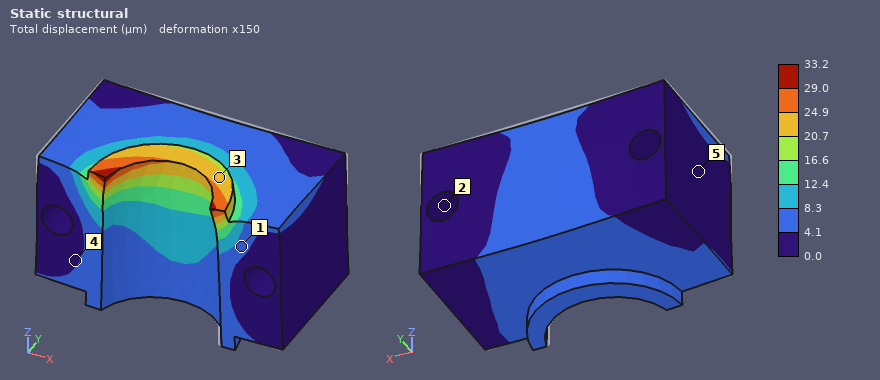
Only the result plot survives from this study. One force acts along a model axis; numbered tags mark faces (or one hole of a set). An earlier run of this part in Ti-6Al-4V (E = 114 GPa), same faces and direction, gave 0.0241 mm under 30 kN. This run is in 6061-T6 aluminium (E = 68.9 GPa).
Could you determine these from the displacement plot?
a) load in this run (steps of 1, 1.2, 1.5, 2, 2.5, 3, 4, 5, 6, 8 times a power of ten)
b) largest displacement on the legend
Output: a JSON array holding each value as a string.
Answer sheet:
["25 kN", "33.2 µm"]
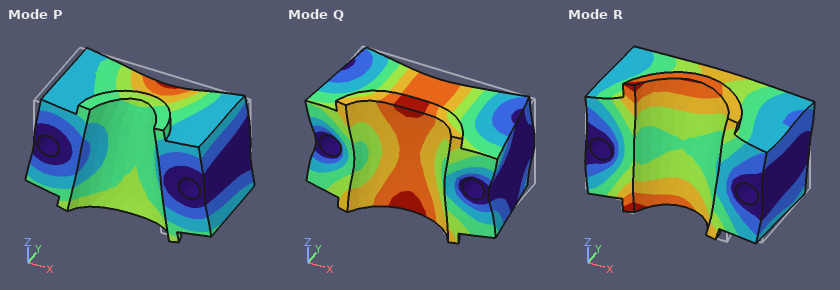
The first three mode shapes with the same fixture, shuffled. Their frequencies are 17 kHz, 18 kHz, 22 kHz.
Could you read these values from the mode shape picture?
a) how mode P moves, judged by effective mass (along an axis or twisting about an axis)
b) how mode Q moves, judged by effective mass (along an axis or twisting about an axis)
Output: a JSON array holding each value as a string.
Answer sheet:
["along Z", "along Y"]
